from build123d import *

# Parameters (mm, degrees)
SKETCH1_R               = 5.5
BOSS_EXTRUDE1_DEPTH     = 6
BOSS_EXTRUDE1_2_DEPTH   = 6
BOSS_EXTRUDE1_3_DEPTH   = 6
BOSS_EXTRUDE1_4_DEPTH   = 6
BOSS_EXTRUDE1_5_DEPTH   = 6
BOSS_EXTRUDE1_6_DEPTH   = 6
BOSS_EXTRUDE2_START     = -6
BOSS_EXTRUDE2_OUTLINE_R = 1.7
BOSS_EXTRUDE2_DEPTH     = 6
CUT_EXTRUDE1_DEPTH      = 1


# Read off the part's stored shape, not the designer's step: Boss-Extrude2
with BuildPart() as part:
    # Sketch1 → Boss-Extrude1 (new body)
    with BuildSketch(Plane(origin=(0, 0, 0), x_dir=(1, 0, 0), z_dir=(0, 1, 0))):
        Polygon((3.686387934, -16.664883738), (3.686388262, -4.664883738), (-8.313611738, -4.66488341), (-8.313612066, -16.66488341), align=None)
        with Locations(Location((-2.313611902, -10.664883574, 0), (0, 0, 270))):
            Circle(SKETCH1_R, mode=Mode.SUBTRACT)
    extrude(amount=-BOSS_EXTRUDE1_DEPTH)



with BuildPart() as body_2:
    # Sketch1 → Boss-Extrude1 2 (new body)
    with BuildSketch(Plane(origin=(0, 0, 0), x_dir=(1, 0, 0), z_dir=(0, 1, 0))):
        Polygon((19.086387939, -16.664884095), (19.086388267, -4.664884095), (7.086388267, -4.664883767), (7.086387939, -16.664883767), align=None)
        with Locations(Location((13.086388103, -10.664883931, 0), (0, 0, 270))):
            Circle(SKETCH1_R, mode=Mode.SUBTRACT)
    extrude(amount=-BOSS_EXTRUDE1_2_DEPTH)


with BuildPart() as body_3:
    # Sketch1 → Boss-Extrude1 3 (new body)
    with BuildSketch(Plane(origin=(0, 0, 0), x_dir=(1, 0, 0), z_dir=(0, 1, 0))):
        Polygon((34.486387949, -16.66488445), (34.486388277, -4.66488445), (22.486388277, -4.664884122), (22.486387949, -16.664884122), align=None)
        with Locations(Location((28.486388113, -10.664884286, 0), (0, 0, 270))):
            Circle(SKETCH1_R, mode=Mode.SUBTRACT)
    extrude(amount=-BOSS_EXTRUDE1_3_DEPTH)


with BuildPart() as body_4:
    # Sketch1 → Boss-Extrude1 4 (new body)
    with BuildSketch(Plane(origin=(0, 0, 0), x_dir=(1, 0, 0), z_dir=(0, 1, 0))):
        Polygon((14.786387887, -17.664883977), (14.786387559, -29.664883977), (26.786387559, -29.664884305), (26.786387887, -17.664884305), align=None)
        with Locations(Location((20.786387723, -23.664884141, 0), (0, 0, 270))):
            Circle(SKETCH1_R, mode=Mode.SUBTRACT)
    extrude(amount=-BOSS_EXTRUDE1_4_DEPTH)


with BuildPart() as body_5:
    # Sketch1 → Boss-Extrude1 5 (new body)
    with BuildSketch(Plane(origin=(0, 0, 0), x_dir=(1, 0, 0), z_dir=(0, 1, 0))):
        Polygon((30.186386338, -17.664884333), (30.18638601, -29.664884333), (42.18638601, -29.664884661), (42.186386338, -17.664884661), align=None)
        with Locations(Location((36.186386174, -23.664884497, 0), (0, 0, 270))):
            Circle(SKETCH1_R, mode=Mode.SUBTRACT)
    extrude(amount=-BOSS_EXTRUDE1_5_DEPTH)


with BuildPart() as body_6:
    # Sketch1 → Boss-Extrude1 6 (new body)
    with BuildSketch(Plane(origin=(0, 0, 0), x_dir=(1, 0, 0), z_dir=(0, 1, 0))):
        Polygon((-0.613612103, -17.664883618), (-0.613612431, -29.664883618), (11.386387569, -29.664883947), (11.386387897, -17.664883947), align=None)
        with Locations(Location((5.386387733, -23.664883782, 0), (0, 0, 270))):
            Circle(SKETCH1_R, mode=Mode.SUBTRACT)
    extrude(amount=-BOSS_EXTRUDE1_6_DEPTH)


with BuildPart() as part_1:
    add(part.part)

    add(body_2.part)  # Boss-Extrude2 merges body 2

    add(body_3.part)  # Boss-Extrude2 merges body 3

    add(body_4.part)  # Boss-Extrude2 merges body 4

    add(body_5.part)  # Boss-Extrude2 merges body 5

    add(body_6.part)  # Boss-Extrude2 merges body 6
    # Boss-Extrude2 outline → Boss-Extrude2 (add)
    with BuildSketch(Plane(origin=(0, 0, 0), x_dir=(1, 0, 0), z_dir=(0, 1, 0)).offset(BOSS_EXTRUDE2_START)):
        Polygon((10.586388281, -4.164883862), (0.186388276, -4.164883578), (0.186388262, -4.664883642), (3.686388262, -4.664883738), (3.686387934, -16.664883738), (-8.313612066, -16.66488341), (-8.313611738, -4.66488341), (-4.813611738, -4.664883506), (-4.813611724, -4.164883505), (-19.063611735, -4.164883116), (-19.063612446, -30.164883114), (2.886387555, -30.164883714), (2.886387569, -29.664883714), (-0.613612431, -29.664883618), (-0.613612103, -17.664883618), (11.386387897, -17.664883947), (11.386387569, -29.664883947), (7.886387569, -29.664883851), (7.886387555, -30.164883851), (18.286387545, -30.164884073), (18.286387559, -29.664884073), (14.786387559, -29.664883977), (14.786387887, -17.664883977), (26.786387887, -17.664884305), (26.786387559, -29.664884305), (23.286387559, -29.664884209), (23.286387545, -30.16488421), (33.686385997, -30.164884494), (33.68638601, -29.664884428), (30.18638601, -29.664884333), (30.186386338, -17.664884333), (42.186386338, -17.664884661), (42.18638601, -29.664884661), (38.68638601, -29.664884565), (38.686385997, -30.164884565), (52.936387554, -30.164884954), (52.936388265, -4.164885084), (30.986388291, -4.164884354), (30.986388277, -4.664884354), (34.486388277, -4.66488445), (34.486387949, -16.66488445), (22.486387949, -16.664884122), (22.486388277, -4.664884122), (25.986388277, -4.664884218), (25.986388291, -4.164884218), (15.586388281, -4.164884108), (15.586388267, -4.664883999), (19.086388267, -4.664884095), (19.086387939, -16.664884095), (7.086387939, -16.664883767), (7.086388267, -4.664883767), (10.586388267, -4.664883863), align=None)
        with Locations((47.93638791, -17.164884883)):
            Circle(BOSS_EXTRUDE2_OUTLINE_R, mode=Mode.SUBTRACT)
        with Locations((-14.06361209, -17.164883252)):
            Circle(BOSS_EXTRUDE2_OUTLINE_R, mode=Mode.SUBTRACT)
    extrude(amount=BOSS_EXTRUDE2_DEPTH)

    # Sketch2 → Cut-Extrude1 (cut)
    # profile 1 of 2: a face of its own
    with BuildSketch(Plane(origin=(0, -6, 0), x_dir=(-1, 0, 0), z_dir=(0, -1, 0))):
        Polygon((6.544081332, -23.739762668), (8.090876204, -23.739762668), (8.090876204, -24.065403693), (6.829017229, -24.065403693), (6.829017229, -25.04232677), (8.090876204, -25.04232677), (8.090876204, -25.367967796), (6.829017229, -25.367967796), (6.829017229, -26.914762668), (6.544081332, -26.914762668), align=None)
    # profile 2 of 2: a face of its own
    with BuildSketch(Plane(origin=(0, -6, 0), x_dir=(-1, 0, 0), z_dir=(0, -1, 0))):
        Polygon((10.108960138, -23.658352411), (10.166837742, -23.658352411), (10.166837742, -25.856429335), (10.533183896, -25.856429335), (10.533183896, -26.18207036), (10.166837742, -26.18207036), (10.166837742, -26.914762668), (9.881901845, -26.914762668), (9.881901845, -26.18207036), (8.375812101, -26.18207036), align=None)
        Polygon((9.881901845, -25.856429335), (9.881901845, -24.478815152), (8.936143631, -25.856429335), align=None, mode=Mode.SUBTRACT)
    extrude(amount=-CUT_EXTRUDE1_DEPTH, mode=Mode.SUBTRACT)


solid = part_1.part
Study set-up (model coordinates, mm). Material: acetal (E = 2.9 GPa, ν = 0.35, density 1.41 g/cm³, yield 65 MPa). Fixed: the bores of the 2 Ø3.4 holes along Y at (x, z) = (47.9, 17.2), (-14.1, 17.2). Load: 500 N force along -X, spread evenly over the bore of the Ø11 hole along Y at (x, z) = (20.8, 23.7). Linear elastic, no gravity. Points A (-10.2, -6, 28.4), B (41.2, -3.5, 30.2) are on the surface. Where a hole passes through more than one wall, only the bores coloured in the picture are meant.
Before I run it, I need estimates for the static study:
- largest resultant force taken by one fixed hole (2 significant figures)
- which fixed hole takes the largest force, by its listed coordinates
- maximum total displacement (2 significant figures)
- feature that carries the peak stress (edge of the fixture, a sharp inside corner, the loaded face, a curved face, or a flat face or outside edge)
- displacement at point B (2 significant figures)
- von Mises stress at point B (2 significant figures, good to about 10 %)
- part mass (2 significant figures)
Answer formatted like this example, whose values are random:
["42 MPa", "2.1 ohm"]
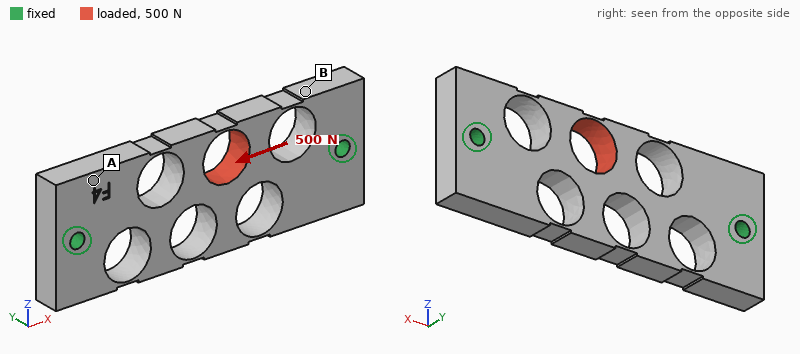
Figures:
["290 N", "(47.9, 17.2)", "0.12 mm", "a curved face", "0.052 mm", "8.2 MPa", "11 g"]
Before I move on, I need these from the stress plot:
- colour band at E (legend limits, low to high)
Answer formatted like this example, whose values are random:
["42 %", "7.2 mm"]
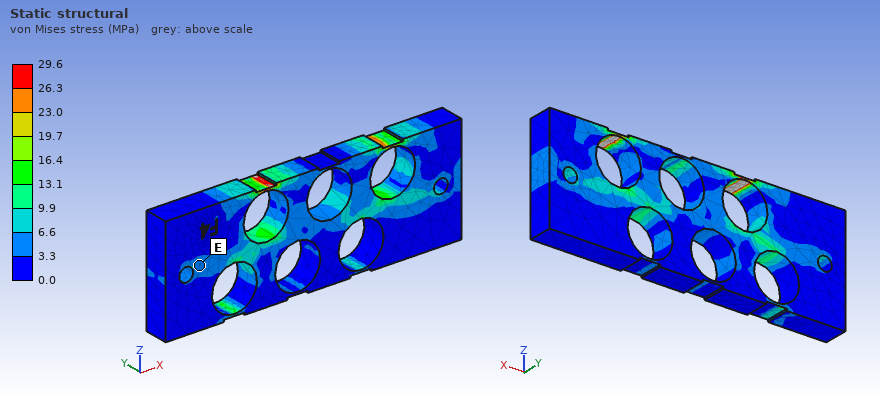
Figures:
["3.3 to 6.6 MPa"]
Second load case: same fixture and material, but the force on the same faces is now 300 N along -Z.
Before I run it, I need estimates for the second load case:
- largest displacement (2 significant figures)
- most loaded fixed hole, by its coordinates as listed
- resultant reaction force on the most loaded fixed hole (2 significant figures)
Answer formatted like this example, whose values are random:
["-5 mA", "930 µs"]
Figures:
["0.29 mm", "(47.9, 17.2)", "170 N"]
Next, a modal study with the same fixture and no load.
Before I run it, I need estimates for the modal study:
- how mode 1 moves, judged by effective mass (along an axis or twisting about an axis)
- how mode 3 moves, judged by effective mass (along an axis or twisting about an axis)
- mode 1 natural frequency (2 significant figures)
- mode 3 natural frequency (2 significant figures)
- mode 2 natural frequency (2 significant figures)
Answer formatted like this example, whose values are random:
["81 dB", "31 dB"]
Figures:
["along Y", "along Z", "1900 Hz", "2800 Hz", "2700 Hz"]
